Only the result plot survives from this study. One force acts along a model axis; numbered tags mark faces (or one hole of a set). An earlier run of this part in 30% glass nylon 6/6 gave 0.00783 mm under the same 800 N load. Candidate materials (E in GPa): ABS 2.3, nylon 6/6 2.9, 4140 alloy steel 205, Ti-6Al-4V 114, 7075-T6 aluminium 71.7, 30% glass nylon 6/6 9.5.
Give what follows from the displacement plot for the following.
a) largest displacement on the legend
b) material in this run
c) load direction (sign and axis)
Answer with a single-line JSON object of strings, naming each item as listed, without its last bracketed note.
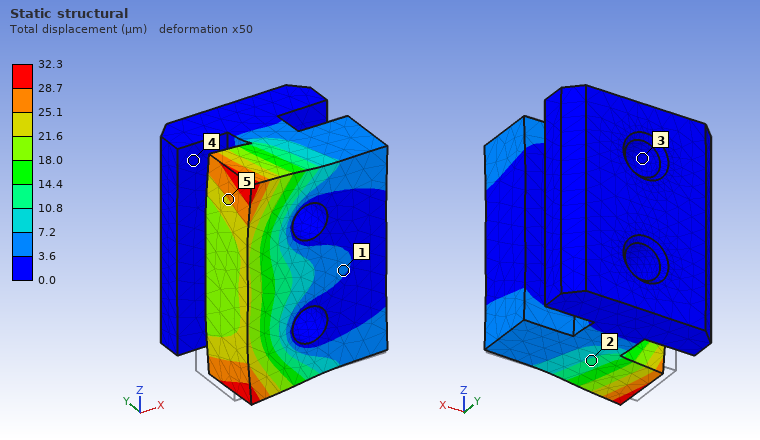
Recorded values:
{"largest displacement on the legend": "32.3 µm", "material in this run": "ABS", "load direction": "+X"}
